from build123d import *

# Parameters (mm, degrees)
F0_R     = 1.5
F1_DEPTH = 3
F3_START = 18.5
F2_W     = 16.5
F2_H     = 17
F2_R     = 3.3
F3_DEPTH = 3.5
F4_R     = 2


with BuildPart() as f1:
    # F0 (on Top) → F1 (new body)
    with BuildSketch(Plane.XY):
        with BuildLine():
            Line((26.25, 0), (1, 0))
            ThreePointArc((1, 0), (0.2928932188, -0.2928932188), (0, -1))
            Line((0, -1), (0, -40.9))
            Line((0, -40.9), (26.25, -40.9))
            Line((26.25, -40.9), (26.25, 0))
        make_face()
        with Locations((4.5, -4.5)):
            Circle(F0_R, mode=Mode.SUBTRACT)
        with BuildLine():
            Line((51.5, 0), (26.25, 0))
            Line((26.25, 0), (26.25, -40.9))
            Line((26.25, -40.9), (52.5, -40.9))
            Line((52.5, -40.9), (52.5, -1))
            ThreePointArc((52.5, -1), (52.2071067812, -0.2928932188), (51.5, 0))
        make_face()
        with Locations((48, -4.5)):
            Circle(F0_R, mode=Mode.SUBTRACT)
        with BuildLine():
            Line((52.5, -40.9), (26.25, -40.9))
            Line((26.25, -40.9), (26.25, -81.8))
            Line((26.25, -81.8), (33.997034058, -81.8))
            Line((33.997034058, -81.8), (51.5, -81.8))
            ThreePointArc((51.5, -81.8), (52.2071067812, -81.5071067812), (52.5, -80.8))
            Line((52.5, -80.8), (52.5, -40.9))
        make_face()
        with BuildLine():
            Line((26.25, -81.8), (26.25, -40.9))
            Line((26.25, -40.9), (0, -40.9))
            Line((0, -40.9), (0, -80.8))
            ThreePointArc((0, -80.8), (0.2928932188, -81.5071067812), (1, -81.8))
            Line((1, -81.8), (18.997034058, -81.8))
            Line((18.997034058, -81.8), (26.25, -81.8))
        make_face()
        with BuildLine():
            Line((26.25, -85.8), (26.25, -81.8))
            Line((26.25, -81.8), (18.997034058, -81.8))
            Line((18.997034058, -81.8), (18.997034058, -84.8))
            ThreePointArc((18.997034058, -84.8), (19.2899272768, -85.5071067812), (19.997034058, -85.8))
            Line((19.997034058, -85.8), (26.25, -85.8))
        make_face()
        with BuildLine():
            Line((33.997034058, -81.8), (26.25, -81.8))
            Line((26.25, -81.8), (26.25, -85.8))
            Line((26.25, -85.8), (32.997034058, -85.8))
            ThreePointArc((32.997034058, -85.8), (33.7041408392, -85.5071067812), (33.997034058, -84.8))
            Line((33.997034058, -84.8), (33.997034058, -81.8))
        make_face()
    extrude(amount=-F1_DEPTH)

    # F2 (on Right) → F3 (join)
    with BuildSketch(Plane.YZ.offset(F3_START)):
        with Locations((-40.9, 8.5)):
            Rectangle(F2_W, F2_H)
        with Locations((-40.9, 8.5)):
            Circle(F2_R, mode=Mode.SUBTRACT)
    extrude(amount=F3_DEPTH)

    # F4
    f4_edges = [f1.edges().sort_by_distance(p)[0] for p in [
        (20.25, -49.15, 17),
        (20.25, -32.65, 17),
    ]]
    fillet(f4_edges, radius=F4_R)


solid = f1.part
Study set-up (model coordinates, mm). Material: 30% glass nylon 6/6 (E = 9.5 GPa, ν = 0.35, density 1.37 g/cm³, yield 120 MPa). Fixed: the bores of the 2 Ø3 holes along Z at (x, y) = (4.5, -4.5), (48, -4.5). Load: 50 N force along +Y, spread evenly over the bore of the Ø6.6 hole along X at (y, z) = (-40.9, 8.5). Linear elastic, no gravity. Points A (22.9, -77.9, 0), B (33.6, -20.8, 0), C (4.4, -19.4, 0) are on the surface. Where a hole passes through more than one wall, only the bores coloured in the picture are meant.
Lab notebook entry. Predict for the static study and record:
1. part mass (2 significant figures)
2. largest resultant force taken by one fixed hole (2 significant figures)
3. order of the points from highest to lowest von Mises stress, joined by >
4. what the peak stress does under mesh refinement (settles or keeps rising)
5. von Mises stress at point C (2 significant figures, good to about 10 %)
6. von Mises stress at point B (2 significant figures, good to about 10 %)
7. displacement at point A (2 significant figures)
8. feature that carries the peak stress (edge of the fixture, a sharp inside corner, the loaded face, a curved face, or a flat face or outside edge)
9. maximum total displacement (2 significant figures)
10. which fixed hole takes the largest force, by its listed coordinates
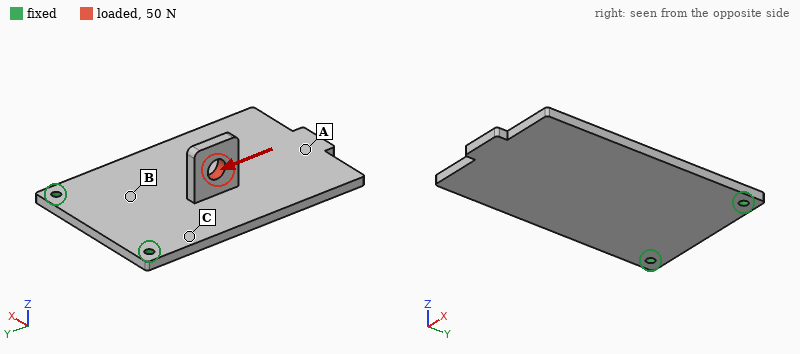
19 g
33 N
C > B > A
keeps rising
7.7 MPa
5.7 MPa
1.0 mm
edge of the fixture
1.2 mm
(4.5, -4.5)
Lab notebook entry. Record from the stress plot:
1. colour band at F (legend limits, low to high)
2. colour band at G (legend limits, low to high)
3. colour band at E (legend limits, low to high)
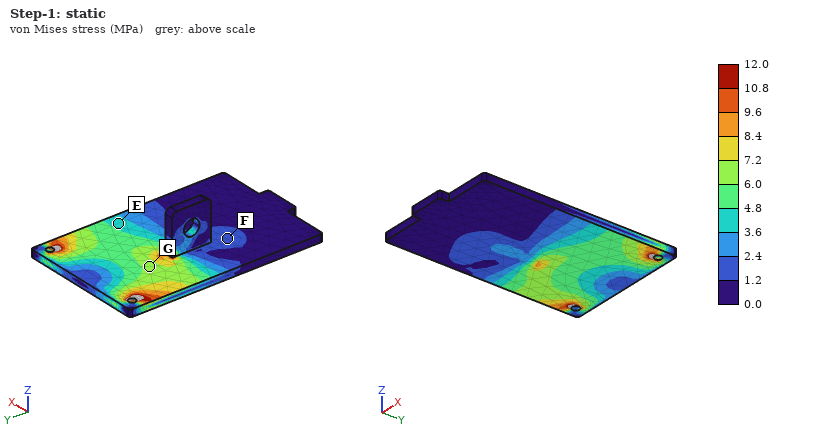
1.2 to 2.4 MPa
6.0 to 7.2 MPa
3.6 to 4.8 MPa
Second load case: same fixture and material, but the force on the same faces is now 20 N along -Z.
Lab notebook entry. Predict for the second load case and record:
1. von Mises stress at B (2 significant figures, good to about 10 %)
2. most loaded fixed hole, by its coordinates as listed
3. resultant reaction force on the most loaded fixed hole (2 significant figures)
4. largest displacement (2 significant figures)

4.7 MPa
(4.5, -4.5)
13 N
1.1 mm
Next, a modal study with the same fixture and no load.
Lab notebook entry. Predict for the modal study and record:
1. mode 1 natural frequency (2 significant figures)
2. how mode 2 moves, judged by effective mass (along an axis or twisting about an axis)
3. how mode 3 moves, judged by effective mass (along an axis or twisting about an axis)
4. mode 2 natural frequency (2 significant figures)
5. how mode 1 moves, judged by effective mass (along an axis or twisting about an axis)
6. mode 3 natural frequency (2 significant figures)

180 Hz
twisting about Y
along Z
700 Hz
along Z
1200 Hz
